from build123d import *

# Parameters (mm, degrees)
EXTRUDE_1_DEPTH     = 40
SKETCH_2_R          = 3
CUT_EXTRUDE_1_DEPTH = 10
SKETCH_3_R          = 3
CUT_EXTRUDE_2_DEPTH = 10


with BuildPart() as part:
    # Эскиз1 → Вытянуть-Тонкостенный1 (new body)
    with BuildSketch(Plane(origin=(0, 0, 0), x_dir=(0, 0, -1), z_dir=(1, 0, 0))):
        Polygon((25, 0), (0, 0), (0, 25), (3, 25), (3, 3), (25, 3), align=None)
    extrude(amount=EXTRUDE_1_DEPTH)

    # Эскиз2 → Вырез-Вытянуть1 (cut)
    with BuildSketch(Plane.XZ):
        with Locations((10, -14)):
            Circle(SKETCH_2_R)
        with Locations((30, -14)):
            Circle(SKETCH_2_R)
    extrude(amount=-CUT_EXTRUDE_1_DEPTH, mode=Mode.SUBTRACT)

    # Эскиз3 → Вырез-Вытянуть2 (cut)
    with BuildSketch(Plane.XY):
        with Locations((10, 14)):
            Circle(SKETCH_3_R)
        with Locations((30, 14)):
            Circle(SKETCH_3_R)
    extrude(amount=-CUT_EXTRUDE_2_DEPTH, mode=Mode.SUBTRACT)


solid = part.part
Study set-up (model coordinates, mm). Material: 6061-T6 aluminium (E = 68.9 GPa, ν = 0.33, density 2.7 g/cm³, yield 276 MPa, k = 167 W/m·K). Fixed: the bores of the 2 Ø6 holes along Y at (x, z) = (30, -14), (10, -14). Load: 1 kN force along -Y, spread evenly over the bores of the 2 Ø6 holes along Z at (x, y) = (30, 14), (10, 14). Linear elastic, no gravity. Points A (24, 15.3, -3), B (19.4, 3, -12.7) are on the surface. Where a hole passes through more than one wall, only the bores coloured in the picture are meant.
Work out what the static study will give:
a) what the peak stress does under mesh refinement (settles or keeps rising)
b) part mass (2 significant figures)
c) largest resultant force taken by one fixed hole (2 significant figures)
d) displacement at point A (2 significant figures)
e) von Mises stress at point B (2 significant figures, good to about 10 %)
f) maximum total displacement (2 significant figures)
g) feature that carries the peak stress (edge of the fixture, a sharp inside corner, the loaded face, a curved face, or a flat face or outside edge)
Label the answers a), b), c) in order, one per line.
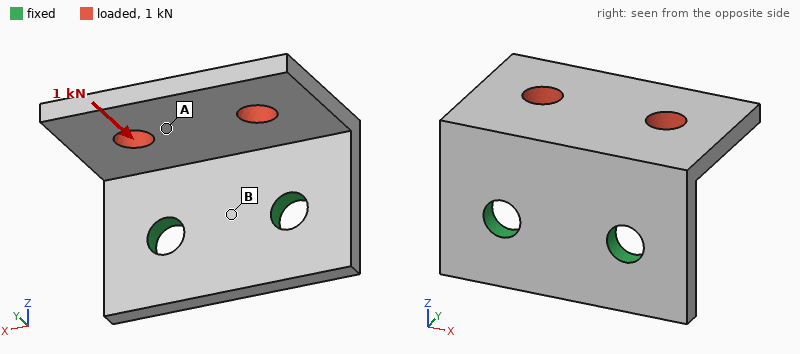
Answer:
a) keeps rising
b) 14 g
c) 500 N
d) 0.14 mm
e) 64 MPa
f) 0.24 mm
g) edge of the fixture
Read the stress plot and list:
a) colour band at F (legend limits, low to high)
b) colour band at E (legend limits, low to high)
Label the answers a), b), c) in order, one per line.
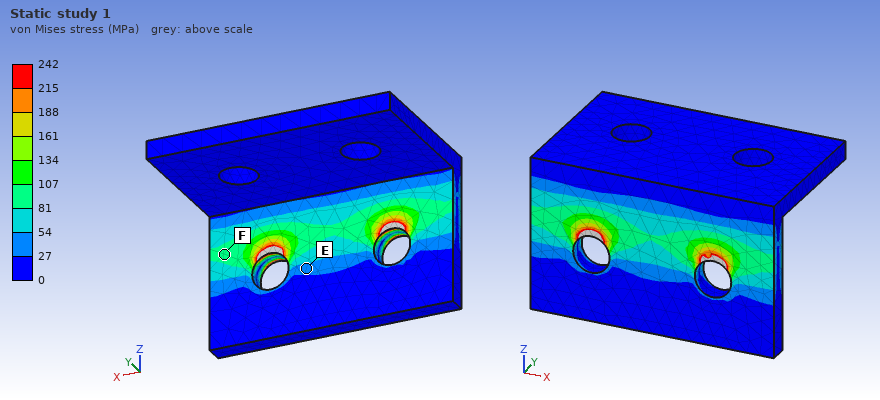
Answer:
a) 81 to 107 MPa
b) 27 to 54 MPa
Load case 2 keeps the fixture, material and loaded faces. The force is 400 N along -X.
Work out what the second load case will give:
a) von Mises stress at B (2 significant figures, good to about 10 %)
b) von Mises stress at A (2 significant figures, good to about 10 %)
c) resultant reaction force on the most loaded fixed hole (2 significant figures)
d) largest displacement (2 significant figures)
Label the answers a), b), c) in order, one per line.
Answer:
a) 8.3 MPa
b) 11 MPa
c) 340 N
d) 57 µm
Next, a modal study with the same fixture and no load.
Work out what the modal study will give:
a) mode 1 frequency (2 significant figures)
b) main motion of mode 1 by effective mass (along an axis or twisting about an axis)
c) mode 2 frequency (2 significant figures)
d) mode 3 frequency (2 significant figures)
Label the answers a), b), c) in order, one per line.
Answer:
a) 2700 Hz
b) along Z
c) 4900 Hz
d) 7600 Hz
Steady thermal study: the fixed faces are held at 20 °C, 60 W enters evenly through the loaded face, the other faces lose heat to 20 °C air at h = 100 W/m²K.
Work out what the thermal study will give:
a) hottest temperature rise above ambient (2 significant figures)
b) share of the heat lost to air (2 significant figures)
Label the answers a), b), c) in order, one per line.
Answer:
a) 68 K
b) 20 %
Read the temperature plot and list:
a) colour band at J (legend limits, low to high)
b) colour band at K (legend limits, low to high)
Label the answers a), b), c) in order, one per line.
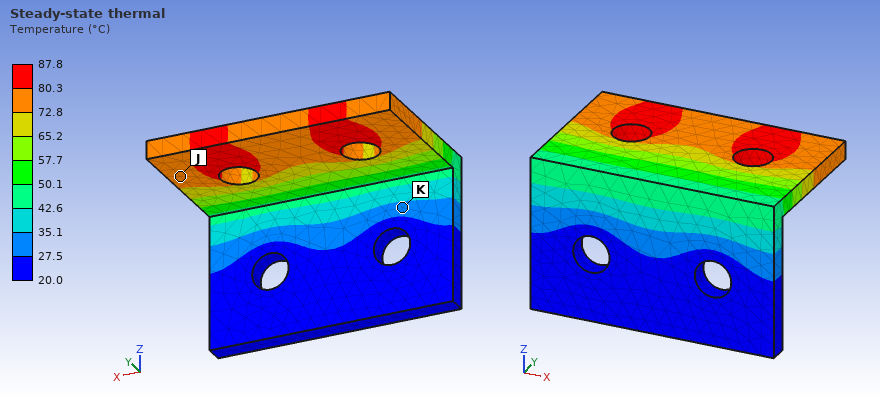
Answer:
a) 72.8 to 80.3 °C
b) 27.5 to 35.1 °C
